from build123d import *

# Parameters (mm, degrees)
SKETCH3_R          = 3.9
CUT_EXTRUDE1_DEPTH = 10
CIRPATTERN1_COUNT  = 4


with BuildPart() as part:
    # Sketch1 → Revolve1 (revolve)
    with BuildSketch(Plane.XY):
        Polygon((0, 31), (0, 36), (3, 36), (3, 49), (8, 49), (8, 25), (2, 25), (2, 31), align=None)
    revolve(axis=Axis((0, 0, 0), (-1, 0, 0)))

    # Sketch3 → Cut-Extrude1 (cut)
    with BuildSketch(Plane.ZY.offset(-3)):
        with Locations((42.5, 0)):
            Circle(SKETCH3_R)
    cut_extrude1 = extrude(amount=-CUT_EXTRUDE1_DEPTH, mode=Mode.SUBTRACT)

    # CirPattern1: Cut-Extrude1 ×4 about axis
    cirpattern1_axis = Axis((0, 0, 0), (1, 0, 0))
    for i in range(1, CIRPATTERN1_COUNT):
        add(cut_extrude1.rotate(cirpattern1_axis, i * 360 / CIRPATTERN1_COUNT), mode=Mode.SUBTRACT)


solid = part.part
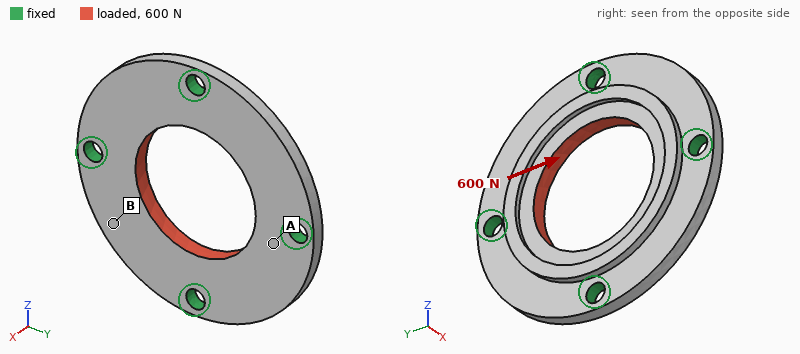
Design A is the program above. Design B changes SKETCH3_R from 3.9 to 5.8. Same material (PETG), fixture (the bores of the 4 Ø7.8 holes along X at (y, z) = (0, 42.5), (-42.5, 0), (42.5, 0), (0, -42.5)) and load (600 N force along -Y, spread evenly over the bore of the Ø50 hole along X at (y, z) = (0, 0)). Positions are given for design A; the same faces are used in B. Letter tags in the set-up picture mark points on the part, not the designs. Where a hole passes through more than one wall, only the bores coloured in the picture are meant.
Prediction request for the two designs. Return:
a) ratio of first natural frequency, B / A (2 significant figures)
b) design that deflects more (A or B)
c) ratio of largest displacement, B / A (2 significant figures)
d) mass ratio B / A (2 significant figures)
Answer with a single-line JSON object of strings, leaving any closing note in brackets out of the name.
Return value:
{"ratio of first natural frequency, B / A": "1.2", "design that deflects more": "A", "ratio of largest displacement, B / A": "0.83", "mass ratio B / A": "0.96"}
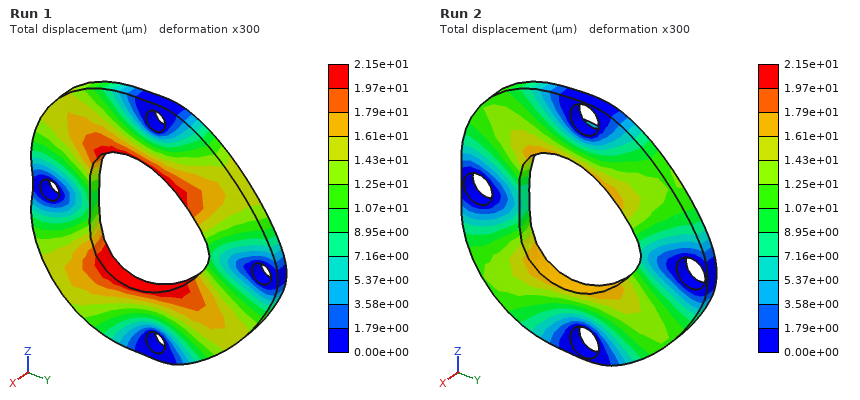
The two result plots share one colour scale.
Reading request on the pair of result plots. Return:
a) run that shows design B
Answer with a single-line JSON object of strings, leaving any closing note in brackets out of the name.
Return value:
{"run that shows design B": "Run 2"}
